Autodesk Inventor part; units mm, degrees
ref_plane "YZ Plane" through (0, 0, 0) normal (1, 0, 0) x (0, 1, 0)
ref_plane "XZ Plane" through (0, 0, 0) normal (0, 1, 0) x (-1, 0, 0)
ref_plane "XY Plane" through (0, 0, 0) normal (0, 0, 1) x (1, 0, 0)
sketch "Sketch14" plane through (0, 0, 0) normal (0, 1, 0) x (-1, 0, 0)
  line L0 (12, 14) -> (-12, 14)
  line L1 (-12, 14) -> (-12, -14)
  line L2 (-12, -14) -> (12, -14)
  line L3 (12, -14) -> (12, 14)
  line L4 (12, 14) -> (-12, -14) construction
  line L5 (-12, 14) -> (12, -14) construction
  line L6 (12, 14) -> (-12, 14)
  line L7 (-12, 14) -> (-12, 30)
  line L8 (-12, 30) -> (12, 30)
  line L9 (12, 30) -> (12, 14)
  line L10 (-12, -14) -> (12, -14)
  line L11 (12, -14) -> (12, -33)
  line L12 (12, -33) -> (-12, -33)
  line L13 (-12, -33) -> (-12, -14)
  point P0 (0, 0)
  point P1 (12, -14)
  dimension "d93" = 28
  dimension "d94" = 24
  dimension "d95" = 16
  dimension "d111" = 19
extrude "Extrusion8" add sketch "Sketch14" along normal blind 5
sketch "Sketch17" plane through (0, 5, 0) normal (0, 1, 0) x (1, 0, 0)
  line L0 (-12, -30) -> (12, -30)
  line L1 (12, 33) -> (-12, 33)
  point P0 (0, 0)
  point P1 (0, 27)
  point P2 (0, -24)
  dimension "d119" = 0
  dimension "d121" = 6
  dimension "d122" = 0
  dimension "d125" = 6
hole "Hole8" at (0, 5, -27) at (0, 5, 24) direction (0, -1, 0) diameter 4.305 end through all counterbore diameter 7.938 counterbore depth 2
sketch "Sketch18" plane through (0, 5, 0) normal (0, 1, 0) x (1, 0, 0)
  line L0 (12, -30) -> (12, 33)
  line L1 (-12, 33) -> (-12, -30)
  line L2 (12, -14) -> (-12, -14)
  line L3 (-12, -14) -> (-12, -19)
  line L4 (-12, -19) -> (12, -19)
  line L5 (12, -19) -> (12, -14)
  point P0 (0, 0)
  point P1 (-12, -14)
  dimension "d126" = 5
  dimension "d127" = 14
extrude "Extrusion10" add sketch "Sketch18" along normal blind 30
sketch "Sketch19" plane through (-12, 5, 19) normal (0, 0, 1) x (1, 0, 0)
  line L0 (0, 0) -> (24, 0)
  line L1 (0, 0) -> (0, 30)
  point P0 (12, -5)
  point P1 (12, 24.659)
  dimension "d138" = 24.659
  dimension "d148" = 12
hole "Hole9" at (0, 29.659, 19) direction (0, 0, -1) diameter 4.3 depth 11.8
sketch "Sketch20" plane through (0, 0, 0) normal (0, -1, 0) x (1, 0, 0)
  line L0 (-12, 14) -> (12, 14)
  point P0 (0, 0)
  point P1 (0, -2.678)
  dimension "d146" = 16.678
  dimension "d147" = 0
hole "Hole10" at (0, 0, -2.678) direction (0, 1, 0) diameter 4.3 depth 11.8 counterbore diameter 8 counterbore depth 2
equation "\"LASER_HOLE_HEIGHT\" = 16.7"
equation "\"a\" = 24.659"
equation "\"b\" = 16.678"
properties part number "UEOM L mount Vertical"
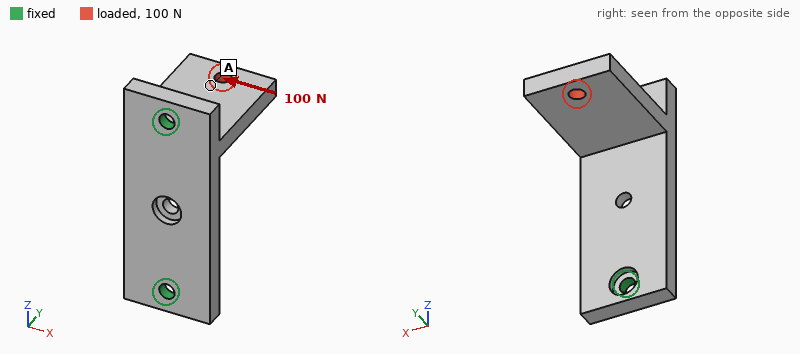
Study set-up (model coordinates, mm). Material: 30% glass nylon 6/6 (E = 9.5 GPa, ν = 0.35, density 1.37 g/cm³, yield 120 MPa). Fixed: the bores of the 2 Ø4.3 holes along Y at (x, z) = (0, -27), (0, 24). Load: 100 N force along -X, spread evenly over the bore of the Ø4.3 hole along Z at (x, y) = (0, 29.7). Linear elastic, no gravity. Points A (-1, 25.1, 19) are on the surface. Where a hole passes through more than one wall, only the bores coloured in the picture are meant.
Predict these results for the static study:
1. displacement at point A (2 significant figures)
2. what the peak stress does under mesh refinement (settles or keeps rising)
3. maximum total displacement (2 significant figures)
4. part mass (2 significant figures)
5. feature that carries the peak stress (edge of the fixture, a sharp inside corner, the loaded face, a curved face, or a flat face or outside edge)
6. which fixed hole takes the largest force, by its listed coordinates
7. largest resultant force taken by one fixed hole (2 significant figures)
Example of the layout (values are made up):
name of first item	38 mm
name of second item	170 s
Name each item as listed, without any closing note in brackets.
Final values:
displacement at point A	0.22 mm
what the peak stress does under mesh refinement	keeps rising
maximum total displacement	0.33 mm
part mass	15 g
feature that carries the peak stress	edge of the fixture
which fixed hole takes the largest force, by its listed coordinates	(0, 24)
largest resultant force taken by one fixed hole	85 N
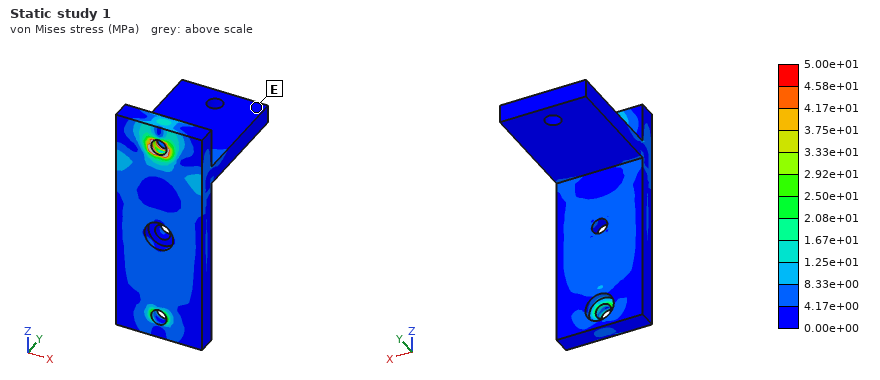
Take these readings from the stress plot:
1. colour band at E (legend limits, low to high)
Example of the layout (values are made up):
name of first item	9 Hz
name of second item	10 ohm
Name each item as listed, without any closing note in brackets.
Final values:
colour band at E	0.00e+00 to 4.17e+00 MPa
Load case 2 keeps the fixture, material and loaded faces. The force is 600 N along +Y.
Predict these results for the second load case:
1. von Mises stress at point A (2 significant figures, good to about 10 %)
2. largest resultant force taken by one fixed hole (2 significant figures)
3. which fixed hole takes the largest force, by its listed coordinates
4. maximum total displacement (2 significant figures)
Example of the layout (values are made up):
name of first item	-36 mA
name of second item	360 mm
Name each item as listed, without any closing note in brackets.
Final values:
von Mises stress at point A	9.5 MPa
largest resultant force taken by one fixed hole	570 N
which fixed hole takes the largest force, by its listed coordinates	(0, 24)
maximum total displacement	0.23 mm
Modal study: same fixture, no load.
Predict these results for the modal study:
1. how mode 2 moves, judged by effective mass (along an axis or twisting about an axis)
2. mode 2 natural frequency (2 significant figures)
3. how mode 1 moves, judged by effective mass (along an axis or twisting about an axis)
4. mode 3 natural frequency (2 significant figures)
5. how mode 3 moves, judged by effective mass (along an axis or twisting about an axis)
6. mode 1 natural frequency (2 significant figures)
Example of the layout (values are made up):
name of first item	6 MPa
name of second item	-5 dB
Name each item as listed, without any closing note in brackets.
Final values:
how mode 2 moves, judged by effective mass	along X
mode 2 natural frequency	1800 Hz
how mode 1 moves, judged by effective mass	along Z
mode 3 natural frequency	4300 Hz
how mode 3 moves, judged by effective mass	along Y
mode 1 natural frequency	1600 Hz
